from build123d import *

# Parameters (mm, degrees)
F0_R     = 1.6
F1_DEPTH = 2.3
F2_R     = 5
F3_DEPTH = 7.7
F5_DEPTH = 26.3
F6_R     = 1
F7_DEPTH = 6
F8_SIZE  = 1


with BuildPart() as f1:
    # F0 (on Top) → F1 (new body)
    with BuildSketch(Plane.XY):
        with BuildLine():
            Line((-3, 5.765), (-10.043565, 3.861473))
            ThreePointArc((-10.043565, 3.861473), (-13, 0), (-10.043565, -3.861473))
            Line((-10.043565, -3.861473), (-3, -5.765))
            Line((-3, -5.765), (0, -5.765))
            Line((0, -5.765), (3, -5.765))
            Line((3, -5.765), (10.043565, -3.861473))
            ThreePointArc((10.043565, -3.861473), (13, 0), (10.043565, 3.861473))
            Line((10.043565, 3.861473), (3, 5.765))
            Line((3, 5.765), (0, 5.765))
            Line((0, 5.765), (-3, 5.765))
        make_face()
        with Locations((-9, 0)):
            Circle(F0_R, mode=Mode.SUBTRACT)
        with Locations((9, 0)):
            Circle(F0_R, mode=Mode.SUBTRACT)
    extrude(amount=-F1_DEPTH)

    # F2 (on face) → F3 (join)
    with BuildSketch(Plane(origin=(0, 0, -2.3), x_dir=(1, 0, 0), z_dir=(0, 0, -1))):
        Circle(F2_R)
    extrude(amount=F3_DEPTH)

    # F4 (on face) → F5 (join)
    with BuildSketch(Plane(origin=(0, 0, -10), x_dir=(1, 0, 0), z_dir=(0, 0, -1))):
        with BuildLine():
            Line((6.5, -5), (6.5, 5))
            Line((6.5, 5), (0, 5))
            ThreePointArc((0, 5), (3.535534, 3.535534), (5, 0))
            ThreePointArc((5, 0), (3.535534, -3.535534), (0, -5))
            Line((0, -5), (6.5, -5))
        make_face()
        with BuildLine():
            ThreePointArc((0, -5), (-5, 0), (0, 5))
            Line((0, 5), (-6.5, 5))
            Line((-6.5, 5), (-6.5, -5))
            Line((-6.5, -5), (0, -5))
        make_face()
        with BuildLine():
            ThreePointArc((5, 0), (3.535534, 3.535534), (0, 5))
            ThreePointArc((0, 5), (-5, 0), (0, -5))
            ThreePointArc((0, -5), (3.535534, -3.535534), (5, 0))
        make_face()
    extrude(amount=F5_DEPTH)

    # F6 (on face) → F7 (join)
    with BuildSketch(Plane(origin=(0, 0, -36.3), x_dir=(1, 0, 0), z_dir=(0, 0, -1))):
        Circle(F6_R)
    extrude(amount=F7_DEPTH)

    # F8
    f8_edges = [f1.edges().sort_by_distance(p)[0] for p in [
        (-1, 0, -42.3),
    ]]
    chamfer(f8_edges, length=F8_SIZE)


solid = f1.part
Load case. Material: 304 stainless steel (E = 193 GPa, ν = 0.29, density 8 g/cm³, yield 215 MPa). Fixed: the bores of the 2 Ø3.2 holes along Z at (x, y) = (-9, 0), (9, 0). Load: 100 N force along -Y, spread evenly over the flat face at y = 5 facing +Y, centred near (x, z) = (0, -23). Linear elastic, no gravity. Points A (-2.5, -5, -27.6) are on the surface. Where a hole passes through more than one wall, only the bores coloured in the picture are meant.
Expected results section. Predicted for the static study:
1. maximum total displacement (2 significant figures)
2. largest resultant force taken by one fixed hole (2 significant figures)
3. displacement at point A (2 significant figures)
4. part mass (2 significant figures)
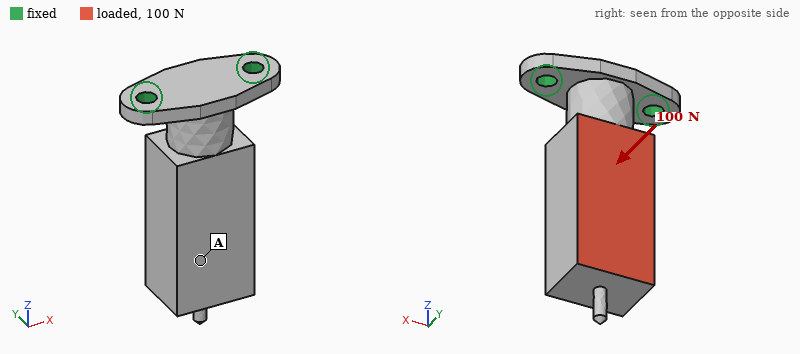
64 µm
50 N
41 µm
36 g
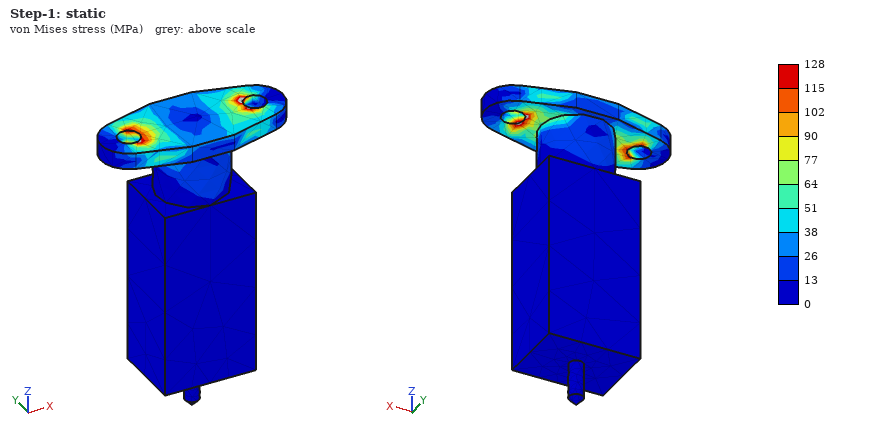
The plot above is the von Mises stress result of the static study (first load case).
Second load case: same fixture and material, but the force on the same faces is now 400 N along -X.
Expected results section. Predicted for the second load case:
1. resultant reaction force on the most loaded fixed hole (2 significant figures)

720 N
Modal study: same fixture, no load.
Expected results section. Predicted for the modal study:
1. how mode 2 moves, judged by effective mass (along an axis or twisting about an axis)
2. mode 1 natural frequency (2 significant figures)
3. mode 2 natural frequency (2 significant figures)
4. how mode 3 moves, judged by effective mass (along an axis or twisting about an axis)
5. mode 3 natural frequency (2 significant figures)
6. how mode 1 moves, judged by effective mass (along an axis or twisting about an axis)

along X
1500 Hz
3200 Hz
along Z
13 kHz
along Y
